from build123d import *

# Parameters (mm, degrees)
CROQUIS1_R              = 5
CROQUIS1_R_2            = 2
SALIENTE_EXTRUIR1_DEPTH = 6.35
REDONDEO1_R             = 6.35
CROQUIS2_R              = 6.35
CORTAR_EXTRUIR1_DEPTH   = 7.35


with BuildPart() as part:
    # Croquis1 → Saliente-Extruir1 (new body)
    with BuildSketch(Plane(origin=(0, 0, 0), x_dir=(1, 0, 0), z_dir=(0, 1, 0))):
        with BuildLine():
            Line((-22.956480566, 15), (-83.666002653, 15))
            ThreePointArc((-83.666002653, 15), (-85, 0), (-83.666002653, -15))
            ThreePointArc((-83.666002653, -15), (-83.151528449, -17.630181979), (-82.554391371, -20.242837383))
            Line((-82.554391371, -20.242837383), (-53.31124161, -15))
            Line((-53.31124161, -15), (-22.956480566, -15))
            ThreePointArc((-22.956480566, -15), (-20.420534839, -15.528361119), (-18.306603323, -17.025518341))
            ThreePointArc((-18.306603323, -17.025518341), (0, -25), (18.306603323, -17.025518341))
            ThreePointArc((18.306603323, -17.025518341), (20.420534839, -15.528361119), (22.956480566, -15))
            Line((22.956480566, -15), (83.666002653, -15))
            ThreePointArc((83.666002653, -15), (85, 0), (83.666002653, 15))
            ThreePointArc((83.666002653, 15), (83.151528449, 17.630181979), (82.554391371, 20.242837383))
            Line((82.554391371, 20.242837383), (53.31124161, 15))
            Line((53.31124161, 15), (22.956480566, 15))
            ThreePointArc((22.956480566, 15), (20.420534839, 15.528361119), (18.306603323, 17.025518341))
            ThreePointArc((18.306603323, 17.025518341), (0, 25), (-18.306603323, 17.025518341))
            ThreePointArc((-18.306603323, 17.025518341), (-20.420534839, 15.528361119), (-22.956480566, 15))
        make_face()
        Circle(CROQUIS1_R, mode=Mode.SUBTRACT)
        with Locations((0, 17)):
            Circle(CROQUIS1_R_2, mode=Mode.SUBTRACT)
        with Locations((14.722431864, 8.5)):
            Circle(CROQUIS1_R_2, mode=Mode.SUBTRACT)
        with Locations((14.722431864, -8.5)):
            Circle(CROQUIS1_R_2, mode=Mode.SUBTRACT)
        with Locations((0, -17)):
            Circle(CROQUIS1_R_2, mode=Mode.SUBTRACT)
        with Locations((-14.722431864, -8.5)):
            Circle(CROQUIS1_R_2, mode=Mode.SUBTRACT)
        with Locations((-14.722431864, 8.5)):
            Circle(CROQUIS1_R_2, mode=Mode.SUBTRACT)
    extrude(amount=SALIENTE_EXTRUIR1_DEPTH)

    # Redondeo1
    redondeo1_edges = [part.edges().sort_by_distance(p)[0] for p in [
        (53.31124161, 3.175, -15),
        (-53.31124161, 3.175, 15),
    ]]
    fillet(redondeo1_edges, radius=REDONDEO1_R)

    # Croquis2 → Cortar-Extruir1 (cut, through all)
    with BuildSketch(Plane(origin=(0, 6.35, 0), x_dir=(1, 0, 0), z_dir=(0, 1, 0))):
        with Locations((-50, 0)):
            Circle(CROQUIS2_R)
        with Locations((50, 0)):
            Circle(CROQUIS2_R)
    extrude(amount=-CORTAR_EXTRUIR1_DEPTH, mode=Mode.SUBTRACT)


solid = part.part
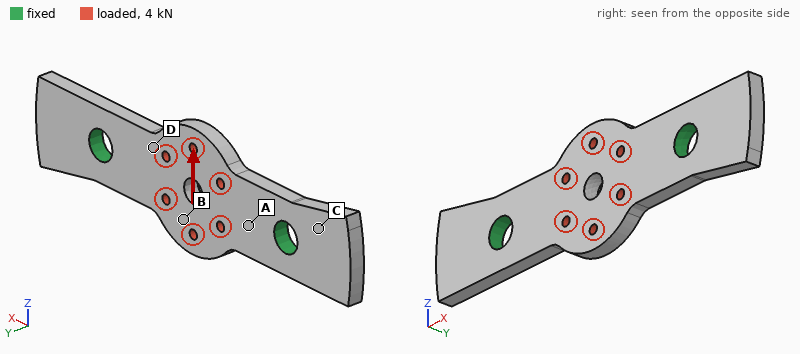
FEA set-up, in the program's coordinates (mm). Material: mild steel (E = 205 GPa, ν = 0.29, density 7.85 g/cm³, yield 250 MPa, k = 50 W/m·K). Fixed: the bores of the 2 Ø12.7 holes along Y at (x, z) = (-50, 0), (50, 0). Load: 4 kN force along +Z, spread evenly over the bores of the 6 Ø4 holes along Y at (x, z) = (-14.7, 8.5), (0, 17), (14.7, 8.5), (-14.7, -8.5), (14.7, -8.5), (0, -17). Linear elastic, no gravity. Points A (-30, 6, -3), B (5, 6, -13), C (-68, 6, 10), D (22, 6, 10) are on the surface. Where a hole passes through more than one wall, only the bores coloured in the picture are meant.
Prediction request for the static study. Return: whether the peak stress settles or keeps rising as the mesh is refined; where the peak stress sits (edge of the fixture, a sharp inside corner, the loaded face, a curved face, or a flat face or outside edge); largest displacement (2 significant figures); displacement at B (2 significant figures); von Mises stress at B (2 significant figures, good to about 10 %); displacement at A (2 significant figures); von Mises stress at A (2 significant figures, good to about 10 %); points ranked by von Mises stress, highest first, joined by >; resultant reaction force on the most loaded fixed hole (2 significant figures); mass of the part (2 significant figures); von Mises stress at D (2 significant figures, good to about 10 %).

keeps rising
edge of the fixture
9.6 µm
9.3 µm
13 MPa
4.9 µm
25 MPa
A > D > B > C
2.0 kN
270 g
20 MPa
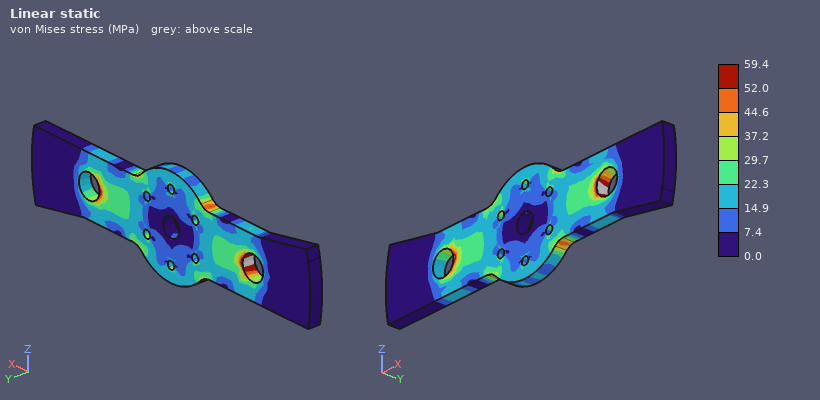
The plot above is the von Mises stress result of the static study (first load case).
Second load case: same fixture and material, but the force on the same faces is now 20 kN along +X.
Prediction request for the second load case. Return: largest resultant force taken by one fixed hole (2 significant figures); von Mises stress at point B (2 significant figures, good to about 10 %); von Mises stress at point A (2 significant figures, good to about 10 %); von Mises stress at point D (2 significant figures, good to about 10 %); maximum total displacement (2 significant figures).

10 kN
19 MPa
55 MPa
52 MPa
11 µm
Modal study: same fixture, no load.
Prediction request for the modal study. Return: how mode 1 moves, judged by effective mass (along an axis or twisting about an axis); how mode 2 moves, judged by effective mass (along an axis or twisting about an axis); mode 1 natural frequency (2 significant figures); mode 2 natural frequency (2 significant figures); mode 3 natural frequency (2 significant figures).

along Y
twisting about X
3400 Hz
4500 Hz
5300 Hz
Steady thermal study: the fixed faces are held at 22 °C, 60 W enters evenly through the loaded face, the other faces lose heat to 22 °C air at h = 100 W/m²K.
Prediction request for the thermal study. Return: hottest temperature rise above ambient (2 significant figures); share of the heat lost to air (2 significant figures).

66 K
52 %
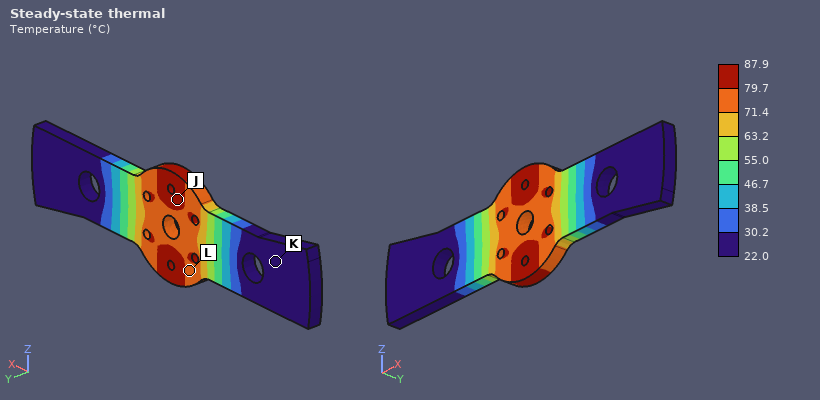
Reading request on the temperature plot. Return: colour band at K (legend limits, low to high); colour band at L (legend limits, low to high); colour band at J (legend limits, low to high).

22.0 to 30.2 °C
71.4 to 79.7 °C
79.7 to 87.9 °C
